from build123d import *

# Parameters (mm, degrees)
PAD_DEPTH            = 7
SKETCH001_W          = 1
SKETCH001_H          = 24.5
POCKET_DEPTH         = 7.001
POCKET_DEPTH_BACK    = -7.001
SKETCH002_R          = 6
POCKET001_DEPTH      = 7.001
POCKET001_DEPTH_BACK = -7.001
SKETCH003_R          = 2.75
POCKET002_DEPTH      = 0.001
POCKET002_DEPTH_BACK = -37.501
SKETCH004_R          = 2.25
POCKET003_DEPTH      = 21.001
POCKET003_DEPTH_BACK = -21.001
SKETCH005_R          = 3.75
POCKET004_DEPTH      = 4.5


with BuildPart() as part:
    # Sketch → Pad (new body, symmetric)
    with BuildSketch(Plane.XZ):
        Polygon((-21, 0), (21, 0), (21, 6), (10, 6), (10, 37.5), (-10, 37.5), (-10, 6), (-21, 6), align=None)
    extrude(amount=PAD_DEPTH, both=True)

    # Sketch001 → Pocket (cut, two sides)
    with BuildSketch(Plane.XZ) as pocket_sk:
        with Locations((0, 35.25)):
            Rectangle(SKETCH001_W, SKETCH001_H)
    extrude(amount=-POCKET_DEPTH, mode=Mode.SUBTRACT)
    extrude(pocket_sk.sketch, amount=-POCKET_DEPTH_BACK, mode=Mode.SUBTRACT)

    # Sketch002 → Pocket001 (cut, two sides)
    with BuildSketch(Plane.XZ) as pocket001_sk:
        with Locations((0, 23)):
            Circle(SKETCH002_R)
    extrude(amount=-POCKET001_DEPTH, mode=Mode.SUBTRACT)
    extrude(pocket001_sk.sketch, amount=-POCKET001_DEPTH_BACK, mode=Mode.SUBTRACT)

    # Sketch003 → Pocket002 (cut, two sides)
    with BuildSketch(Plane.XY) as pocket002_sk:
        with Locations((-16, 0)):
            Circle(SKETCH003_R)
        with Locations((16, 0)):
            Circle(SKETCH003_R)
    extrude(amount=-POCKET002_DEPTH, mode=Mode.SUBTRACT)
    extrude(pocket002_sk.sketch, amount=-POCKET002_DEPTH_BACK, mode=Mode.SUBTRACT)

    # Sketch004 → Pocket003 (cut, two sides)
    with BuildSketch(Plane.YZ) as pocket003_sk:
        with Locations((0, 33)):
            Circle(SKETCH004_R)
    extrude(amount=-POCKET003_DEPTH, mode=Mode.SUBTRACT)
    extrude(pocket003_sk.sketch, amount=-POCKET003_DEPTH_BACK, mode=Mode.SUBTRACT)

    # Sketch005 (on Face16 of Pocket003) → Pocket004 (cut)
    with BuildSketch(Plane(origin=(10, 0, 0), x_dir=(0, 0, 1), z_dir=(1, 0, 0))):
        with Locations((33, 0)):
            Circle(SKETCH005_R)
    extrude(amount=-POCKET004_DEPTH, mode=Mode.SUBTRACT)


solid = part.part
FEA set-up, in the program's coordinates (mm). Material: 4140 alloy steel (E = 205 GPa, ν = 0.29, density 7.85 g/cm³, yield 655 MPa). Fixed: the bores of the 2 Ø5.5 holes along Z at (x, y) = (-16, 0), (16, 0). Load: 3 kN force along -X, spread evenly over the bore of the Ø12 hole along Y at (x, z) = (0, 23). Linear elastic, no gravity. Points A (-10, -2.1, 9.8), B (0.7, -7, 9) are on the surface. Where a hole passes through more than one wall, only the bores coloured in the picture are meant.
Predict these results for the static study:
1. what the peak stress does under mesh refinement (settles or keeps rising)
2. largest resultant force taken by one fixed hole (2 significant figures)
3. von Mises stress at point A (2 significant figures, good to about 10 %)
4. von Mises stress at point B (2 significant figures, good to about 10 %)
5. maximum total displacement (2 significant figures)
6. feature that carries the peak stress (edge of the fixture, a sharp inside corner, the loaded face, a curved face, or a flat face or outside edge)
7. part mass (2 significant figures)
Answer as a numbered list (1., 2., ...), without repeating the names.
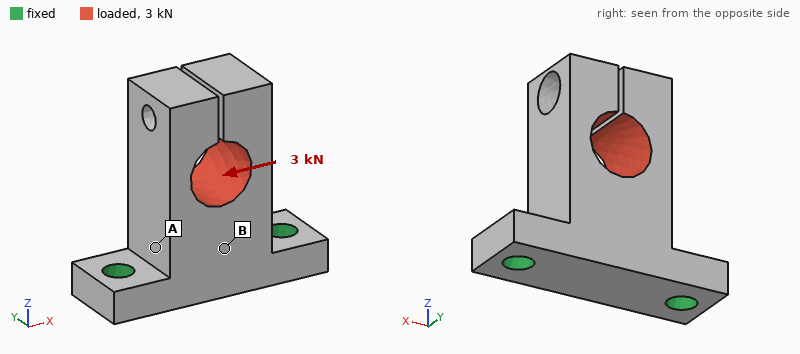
1. keeps rising
2. 2.9 kN
3. 62 MPa
4. 22 MPa
5. 55 µm
6. edge of the fixture
7. 78 g
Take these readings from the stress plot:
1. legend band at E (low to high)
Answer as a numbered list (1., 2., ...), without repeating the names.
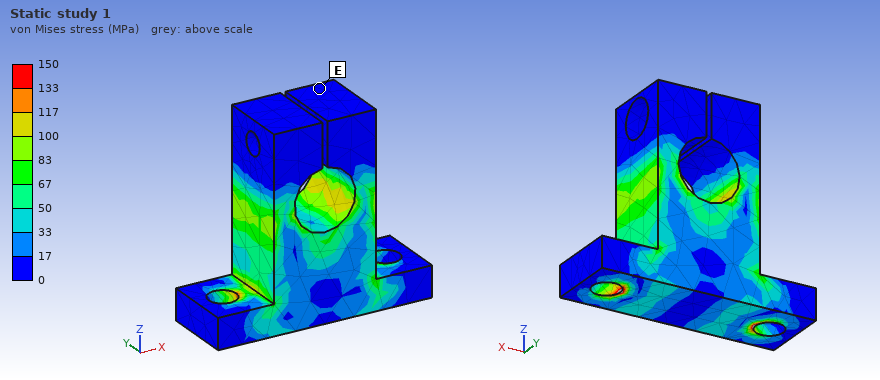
1. 0 to 17 MPa
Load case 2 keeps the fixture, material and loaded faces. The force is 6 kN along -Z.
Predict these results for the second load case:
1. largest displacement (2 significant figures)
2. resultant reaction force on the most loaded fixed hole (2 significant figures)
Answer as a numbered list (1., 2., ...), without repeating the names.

1. 56 µm
2. 3.2 kN
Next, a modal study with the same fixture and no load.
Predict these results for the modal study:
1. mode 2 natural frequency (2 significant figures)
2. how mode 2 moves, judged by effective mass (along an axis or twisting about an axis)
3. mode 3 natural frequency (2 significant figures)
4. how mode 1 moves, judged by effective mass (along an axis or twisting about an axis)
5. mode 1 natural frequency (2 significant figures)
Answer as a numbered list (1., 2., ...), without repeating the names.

1. 5600 Hz
2. along X
3. 6100 Hz
4. along Y
5. 4500 Hz
